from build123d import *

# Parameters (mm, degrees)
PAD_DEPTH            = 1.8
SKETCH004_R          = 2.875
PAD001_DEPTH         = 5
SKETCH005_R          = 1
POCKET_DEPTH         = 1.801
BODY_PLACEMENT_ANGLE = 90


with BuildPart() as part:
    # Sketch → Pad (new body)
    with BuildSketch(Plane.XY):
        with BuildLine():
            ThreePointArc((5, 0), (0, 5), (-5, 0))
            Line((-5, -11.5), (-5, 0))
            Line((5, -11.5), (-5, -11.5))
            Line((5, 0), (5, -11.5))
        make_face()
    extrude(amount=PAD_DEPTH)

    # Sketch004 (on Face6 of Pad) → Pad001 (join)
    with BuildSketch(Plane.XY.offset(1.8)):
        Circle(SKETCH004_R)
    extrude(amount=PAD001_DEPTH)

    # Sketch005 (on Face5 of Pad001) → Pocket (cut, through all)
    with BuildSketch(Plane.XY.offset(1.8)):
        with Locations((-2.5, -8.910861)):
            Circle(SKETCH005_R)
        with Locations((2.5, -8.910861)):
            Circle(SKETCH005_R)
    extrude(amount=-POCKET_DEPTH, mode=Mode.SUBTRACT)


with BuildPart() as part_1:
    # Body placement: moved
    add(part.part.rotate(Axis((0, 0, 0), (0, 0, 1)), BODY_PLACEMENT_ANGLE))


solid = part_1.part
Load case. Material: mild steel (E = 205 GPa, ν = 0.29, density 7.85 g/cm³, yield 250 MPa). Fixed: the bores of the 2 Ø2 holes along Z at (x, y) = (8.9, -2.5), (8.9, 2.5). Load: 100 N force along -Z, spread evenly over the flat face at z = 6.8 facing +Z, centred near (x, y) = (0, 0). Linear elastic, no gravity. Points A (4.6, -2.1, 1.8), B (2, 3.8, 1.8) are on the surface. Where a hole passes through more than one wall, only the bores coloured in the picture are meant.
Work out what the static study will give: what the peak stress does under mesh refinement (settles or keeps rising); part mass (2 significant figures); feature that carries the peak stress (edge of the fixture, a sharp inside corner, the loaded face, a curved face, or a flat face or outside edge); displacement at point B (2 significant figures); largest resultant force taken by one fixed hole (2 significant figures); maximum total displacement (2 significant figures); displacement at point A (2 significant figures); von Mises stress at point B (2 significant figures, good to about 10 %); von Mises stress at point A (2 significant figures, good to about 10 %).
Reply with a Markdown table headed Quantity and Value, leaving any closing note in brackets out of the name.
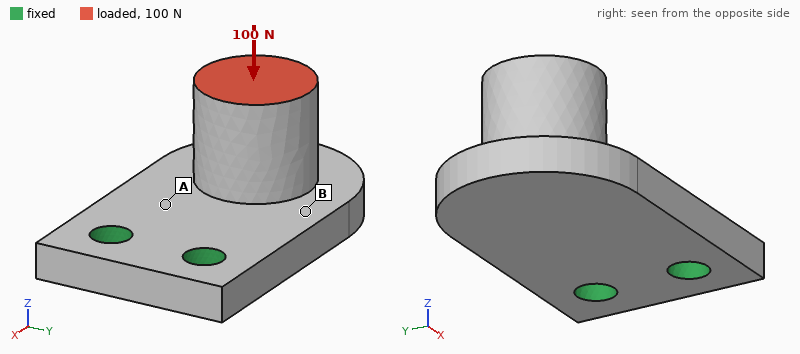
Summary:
| Quantity | Value |
|---|---|
| what the peak stress does under mesh refinement | keeps rising |
| part mass | 3.1 g |
| feature that carries the peak stress | edge of the fixture |
| displacement at point B | 13 µm |
| largest resultant force taken by one fixed hole | 50 N |
| maximum total displacement | 37 µm |
| displacement at point A | 5.8 µm |
| von Mises stress at point B | 33 MPa |
| von Mises stress at point A | 79 MPa |
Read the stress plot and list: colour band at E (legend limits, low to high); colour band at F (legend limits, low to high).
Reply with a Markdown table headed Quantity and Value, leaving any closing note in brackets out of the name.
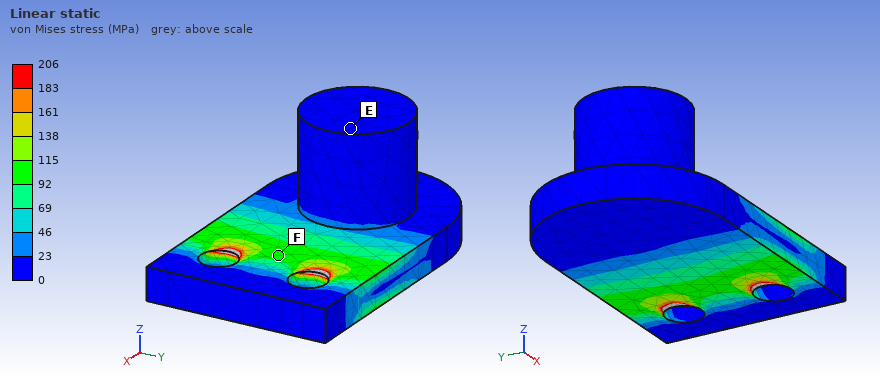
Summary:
| Quantity | Value |
|---|---|
| colour band at E | 0 to 23 MPa |
| colour band at F | 92 to 115 MPa |
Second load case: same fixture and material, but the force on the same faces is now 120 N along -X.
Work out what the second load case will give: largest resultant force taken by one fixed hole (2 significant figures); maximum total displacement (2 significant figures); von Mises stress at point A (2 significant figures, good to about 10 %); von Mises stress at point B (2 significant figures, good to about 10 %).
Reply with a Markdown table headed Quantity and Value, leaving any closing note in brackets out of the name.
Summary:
| Quantity | Value |
|---|---|
| largest resultant force taken by one fixed hole | 62 N |
| maximum total displacement | 48 µm |
| von Mises stress at point A | 130 MPa |
| von Mises stress at point B | 85 MPa |
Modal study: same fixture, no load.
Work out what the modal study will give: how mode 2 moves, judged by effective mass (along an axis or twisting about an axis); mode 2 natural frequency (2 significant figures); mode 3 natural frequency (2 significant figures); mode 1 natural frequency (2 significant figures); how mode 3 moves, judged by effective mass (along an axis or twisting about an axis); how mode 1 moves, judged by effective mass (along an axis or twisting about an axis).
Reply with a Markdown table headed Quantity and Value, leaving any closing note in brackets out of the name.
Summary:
| Quantity | Value |
|---|---|
| how mode 2 moves, judged by effective mass | along Y |
| mode 2 natural frequency | 17 kHz |
| mode 3 natural frequency | 32 kHz |
| mode 1 natural frequency | 6700 Hz |
| how mode 3 moves, judged by effective mass | along Y |
| how mode 1 moves, judged by effective mass | along Z |
